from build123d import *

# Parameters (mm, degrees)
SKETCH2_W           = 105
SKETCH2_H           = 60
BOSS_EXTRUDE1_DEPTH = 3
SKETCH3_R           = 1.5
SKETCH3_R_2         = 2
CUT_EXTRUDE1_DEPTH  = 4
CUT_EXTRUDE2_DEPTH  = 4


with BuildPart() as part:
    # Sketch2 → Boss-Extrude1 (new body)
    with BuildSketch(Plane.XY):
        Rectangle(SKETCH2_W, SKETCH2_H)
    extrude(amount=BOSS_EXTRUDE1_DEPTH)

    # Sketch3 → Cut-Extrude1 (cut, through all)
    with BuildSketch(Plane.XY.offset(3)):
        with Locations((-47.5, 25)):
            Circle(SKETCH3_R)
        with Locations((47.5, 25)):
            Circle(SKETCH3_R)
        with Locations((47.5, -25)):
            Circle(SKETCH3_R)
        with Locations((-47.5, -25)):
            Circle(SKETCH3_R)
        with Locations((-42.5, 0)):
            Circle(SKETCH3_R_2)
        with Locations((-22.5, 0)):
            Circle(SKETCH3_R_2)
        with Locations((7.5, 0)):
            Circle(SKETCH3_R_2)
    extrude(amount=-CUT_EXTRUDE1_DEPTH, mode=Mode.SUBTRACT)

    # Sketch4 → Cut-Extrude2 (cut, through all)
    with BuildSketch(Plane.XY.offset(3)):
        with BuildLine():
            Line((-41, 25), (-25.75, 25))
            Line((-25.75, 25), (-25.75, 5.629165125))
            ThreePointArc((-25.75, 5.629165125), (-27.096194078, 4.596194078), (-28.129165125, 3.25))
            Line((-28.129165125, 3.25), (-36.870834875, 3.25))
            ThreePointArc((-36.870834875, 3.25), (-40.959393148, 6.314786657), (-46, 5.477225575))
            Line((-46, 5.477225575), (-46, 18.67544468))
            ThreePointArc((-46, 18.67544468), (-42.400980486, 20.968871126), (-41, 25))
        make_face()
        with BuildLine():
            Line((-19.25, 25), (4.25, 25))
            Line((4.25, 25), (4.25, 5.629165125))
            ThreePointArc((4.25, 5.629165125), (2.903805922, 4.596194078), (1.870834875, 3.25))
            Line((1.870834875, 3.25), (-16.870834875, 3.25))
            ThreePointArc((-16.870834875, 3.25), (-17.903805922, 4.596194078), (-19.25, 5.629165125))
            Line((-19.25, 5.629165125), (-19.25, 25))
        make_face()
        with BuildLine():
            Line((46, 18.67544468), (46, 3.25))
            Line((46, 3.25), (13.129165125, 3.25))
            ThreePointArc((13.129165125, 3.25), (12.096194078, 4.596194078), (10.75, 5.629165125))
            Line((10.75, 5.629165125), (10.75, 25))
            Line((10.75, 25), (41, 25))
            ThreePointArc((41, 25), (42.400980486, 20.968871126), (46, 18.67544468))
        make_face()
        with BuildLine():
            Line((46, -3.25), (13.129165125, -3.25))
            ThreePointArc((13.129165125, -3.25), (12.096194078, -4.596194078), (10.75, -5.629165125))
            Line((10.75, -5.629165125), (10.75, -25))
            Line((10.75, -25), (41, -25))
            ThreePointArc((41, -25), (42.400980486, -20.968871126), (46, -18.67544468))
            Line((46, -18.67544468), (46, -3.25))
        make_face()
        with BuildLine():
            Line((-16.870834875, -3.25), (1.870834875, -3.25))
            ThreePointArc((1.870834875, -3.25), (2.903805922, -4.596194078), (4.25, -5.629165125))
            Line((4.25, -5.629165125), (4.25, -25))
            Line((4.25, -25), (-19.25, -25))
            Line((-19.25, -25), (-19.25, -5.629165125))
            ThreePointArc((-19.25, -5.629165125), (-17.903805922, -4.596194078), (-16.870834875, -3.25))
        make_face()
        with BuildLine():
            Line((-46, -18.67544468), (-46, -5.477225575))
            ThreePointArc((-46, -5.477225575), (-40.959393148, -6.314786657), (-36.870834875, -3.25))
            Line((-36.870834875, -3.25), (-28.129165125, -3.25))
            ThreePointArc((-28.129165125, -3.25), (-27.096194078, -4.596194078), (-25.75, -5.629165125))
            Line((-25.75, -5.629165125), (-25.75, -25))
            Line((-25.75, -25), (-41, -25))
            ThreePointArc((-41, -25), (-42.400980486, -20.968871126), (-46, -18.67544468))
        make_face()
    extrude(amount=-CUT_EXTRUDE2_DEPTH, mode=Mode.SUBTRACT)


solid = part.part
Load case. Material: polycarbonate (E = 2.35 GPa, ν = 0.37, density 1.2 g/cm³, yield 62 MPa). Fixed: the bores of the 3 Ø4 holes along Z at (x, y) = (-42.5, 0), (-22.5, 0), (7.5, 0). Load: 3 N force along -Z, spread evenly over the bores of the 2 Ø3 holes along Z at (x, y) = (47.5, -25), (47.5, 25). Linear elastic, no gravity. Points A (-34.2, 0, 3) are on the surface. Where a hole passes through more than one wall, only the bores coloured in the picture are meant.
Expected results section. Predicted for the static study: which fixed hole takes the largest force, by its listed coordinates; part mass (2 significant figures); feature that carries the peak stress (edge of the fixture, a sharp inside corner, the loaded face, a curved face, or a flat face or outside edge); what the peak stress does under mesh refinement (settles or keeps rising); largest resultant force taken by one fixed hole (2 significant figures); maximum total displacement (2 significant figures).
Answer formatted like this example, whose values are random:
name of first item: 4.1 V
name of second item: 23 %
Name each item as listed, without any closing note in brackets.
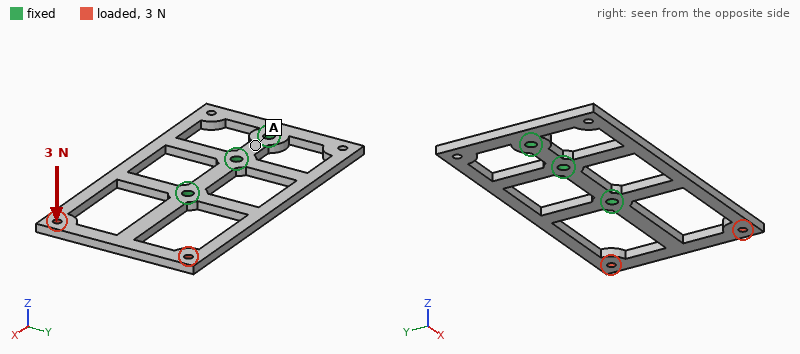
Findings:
which fixed hole takes the largest force, by its listed coordinates: (7.5, 0)
part mass: 11 g
feature that carries the peak stress: edge of the fixture
what the peak stress does under mesh refinement: keeps rising
largest resultant force taken by one fixed hole: 3.9 N
maximum total displacement: 1.1 mm
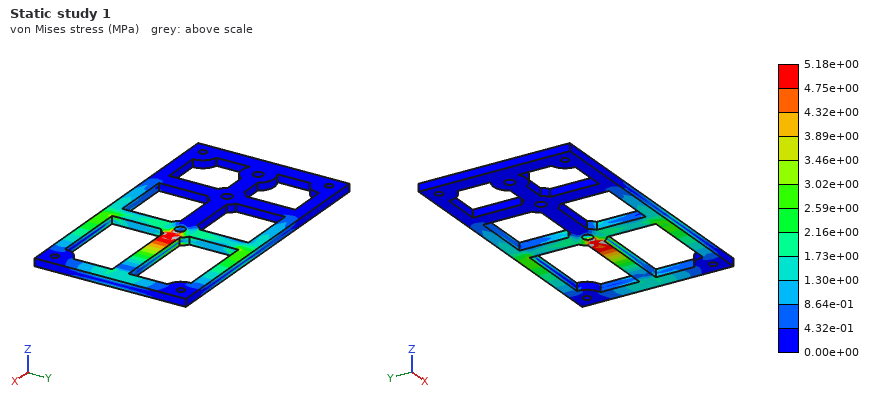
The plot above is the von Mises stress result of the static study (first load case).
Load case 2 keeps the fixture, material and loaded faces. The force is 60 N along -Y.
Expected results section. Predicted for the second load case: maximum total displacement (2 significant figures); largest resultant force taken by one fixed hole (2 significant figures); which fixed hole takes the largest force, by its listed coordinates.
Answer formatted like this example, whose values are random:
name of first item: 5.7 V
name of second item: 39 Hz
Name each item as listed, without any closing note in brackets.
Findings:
maximum total displacement: 1.2 mm
largest resultant force taken by one fixed hole: 86 N
which fixed hole takes the largest force, by its listed coordinates: (7.5, 0)
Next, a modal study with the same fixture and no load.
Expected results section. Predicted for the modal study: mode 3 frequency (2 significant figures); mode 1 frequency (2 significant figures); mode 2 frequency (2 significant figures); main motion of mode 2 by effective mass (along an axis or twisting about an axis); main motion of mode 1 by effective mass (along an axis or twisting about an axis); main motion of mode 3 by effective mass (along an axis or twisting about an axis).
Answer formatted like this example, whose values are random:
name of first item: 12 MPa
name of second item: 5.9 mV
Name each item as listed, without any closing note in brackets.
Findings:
mode 3 frequency: 540 Hz
mode 1 frequency: 200 Hz
mode 2 frequency: 300 Hz
main motion of mode 2 by effective mass: twisting about X
main motion of mode 1 by effective mass: along Z
main motion of mode 3 by effective mass: along Z
